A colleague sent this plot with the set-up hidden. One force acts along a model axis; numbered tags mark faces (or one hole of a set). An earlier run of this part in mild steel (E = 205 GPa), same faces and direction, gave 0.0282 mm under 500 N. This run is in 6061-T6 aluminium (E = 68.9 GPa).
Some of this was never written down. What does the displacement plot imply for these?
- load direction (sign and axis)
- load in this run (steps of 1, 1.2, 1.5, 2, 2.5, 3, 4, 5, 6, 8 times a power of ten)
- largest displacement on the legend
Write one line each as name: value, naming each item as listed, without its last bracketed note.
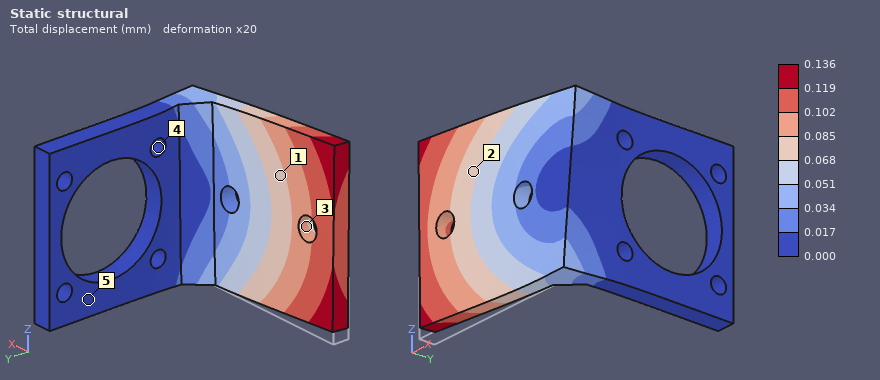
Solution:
load direction: +Z
load in this run: 800 N
largest displacement on the legend: 0.136 mm
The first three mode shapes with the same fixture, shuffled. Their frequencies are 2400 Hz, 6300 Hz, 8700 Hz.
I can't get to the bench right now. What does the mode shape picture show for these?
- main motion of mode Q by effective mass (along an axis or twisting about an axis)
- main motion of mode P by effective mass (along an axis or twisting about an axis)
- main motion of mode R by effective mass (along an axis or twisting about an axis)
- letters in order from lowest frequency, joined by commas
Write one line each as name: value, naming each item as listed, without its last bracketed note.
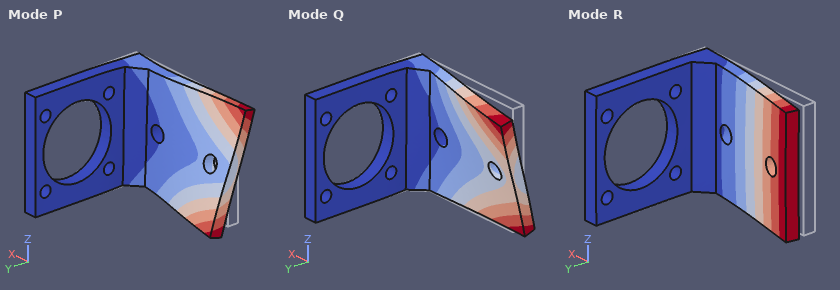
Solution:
main motion of mode Q by effective mass: along Z
main motion of mode P by effective mass: along Z
main motion of mode R by effective mass: along Y
letters in order from lowest frequency, joined by commas: R, Q, P
